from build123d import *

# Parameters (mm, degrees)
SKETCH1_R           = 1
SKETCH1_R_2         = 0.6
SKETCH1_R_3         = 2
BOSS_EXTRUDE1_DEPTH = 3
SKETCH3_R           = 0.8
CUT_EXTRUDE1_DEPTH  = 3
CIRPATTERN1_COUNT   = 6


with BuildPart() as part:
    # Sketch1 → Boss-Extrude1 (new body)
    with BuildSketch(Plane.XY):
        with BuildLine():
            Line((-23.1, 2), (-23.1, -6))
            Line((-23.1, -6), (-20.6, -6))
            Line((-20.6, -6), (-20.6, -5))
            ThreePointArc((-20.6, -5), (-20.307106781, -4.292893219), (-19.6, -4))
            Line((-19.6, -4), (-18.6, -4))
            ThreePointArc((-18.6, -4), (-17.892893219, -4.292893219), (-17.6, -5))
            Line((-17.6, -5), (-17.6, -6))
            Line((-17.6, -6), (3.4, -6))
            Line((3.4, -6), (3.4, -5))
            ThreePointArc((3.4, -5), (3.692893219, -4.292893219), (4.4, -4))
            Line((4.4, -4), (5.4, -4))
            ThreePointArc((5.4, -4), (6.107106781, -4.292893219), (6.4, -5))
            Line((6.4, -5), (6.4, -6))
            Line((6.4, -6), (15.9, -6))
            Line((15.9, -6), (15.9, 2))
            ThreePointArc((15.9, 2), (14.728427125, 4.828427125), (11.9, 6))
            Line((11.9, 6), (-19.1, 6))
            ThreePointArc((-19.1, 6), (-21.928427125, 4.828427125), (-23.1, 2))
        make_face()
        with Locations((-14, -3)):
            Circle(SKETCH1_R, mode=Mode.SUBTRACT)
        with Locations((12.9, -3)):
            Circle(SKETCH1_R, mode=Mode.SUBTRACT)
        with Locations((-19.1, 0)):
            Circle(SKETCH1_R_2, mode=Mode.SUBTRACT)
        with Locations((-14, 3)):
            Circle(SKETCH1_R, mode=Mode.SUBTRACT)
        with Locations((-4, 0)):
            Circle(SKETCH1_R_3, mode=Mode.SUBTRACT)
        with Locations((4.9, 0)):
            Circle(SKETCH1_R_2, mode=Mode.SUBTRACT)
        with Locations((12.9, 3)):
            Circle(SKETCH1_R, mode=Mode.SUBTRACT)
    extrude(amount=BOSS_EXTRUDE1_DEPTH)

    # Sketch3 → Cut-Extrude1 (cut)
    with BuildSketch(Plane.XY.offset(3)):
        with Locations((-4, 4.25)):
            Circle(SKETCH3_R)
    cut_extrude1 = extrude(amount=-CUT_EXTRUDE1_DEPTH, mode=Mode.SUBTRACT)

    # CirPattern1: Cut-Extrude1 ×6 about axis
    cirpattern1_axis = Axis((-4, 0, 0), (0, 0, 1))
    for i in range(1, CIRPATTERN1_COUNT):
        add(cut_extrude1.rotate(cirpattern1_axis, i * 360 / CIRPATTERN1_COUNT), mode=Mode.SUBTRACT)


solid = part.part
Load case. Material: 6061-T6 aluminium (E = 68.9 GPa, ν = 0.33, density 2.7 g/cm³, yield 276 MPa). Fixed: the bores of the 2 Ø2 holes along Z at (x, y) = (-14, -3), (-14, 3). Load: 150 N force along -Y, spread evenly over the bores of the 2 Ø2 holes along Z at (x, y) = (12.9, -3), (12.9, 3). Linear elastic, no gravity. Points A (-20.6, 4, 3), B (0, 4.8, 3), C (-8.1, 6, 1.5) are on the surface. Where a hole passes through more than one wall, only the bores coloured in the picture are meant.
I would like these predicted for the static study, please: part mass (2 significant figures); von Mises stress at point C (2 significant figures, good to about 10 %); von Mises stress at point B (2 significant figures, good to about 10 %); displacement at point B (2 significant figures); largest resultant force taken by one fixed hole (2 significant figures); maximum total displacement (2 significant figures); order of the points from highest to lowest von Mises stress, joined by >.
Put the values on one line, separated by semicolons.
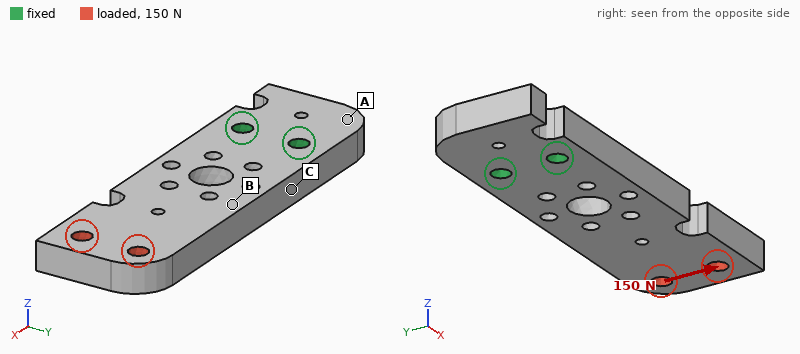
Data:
3.3 g; 49 MPa; 22 MPa; 20 µm; 560 N; 58 µm; C > B > A
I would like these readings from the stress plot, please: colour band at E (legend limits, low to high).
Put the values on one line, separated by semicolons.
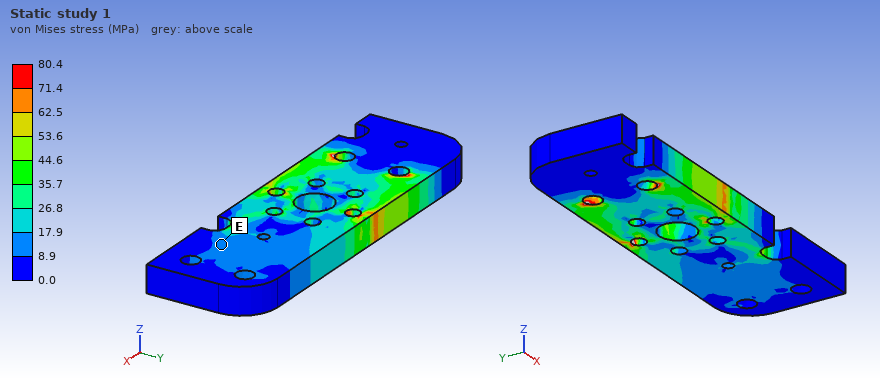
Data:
8.9 to 17.9 MPa
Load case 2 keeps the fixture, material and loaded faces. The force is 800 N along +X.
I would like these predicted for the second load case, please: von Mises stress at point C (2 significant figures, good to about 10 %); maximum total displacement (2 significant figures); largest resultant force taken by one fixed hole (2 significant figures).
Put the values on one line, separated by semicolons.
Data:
27 MPa; 15 µm; 400 N
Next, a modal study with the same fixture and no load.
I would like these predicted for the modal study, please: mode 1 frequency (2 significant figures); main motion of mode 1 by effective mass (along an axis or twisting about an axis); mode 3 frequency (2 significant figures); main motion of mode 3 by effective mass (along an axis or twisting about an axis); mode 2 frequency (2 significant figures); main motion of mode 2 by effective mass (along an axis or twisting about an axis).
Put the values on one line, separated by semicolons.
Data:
2600 Hz; along Z; 12 kHz; twisting about X; 9100 Hz; along Y
